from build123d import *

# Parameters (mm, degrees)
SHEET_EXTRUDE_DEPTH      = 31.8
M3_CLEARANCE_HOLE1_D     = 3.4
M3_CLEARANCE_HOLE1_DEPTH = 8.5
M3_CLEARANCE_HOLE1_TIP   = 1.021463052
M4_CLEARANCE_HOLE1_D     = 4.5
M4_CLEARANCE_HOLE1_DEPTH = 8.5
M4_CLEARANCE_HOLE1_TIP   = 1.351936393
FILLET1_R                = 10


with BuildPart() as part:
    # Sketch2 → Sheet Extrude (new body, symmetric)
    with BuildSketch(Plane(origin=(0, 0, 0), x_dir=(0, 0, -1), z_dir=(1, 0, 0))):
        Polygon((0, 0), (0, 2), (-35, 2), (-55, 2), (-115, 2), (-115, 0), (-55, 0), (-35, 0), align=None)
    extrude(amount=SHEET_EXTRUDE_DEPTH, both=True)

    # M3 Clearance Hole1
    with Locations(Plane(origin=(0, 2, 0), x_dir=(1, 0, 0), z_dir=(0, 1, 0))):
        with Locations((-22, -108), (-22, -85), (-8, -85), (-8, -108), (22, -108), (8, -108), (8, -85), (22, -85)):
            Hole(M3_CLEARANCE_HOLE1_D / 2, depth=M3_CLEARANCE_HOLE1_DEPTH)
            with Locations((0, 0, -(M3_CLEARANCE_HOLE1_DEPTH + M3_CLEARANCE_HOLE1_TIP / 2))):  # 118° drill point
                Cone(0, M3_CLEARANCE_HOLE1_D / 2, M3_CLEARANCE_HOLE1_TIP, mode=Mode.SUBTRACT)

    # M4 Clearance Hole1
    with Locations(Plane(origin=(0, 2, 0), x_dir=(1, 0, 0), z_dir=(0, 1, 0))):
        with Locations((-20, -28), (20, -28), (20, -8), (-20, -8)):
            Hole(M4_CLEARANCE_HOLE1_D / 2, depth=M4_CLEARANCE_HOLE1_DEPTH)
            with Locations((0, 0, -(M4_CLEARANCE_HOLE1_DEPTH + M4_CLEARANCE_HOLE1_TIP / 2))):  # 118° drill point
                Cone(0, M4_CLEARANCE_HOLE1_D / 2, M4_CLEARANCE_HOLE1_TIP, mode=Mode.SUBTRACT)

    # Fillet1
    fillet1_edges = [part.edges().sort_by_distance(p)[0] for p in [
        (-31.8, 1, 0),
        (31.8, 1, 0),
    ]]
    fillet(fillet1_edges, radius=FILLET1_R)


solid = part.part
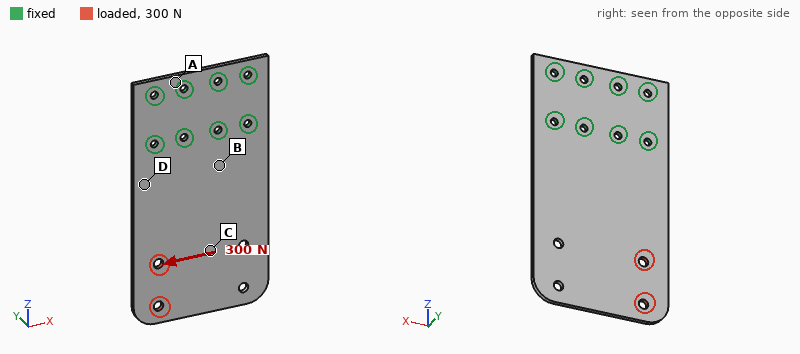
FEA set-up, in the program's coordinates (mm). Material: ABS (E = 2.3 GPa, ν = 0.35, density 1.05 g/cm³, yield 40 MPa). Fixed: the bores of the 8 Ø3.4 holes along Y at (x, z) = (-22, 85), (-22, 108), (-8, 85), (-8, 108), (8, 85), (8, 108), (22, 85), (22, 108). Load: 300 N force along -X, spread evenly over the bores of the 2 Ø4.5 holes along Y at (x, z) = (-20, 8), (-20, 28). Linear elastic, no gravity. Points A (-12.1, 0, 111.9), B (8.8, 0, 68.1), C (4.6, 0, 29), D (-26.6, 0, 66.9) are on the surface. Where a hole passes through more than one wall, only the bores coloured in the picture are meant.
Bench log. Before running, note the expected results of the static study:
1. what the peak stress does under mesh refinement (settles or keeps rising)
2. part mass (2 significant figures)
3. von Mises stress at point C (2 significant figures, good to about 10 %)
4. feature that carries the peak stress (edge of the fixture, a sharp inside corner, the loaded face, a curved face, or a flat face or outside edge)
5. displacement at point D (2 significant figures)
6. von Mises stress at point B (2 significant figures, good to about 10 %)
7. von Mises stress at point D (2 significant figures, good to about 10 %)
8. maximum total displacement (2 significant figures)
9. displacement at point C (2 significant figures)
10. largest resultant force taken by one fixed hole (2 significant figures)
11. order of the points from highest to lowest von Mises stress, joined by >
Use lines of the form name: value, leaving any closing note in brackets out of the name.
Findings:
what the peak stress does under mesh refinement: keeps rising
part mass: 15 g
von Mises stress at point C: 4.9 MPa
feature that carries the peak stress: edge of the fixture
displacement at point D: 0.16 mm
von Mises stress at point B: 6.9 MPa
von Mises stress at point D: 9.2 MPa
maximum total displacement: 0.78 mm
displacement at point C: 0.46 mm
largest resultant force taken by one fixed hole: 340 N
order of the points from highest to lowest von Mises stress, joined by >: D > B > C > A
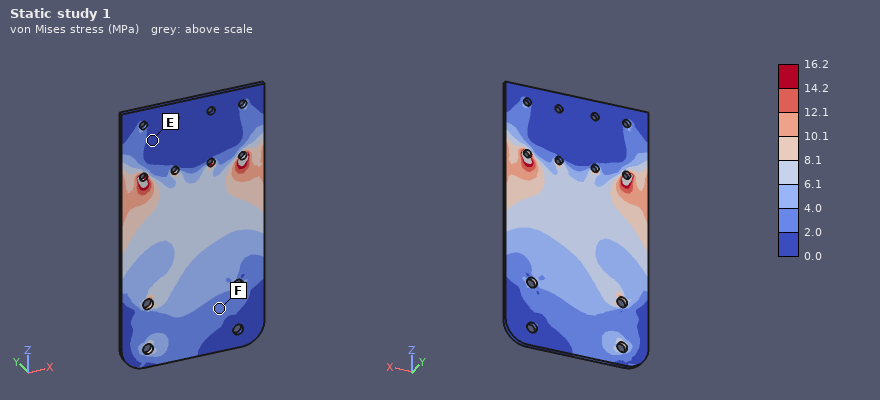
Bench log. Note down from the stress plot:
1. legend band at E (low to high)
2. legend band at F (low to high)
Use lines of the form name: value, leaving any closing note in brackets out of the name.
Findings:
legend band at E: 0.0 to 2.0 MPa
legend band at F: 2.0 to 4.0 MPa
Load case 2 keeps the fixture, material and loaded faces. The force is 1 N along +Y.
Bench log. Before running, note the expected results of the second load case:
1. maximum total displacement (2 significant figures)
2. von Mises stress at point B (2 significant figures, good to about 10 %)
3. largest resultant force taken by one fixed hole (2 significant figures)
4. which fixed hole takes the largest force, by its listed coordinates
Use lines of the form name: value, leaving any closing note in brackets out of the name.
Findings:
maximum total displacement: 1.5 mm
von Mises stress at point B: 1.0 MPa
largest resultant force taken by one fixed hole: 0.64 N
which fixed hole takes the largest force, by its listed coordinates: (-8, 85)
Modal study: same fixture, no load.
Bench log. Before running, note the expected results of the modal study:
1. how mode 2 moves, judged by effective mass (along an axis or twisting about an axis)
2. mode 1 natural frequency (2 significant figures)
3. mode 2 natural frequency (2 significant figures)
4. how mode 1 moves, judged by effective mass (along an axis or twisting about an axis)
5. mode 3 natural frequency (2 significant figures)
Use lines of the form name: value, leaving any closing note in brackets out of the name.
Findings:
how mode 2 moves, judged by effective mass: twisting about Z
mode 1 natural frequency: 71 Hz
mode 2 natural frequency: 210 Hz
how mode 1 moves, judged by effective mass: along Y
mode 3 natural frequency: 430 Hz
